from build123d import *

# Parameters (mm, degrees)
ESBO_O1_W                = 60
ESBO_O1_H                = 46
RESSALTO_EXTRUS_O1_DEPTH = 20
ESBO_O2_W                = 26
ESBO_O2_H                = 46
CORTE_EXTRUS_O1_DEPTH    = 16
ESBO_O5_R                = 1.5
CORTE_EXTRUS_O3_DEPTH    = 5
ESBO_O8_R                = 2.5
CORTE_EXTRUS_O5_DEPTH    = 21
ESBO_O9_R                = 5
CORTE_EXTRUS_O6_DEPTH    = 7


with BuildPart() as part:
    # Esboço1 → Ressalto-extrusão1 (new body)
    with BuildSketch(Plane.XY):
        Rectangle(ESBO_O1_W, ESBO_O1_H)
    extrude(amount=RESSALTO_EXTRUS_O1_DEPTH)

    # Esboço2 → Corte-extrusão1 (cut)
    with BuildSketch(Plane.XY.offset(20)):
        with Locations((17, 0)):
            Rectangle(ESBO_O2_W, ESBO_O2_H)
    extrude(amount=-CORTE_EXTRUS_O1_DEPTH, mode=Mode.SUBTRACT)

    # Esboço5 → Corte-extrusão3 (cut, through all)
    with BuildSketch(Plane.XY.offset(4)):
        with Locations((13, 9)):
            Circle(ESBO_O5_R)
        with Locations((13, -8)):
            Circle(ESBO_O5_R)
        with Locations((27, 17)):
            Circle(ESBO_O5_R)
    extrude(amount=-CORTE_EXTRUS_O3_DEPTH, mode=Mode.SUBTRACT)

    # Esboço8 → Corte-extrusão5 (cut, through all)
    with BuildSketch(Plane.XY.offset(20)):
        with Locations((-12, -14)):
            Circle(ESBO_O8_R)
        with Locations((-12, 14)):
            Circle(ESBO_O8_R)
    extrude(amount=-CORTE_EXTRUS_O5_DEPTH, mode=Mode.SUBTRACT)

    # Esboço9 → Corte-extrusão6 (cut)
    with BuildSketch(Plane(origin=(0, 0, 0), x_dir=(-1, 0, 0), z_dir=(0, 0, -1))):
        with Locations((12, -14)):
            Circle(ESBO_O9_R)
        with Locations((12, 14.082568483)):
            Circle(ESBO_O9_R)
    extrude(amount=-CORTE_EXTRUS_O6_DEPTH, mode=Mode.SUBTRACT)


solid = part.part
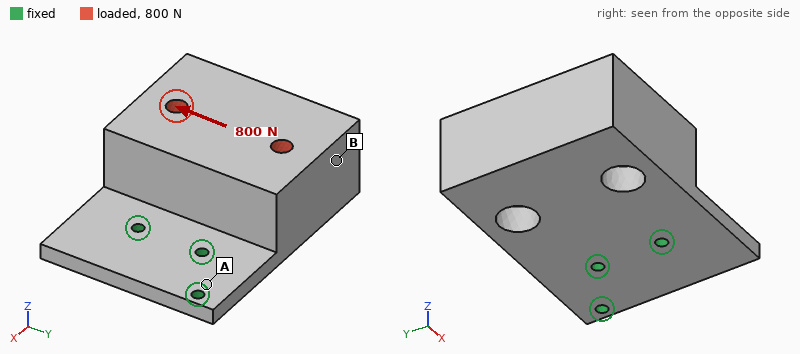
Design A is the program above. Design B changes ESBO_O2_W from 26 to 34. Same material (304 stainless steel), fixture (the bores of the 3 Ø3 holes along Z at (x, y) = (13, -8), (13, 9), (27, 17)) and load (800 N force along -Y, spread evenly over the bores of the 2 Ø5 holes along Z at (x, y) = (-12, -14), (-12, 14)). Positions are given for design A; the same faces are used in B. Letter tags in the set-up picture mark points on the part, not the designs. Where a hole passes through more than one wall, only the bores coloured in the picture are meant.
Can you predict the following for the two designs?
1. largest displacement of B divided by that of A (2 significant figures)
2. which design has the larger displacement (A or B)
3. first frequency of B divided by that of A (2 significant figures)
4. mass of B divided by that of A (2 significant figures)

1.6
B
0.94
0.91
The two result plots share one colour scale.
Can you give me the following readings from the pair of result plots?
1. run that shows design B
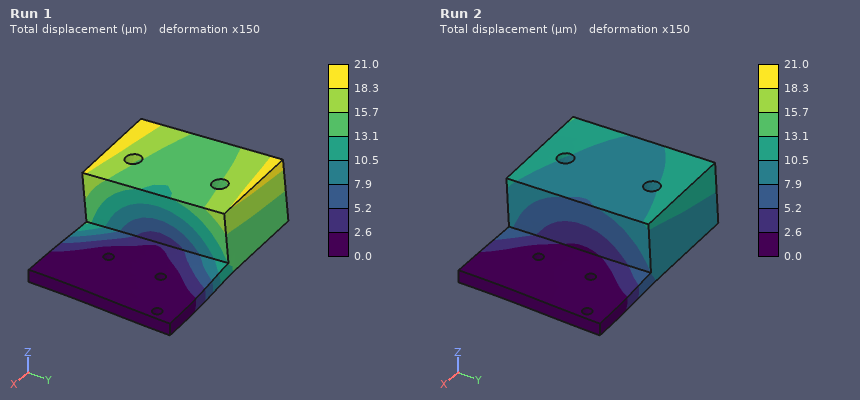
Run 1
